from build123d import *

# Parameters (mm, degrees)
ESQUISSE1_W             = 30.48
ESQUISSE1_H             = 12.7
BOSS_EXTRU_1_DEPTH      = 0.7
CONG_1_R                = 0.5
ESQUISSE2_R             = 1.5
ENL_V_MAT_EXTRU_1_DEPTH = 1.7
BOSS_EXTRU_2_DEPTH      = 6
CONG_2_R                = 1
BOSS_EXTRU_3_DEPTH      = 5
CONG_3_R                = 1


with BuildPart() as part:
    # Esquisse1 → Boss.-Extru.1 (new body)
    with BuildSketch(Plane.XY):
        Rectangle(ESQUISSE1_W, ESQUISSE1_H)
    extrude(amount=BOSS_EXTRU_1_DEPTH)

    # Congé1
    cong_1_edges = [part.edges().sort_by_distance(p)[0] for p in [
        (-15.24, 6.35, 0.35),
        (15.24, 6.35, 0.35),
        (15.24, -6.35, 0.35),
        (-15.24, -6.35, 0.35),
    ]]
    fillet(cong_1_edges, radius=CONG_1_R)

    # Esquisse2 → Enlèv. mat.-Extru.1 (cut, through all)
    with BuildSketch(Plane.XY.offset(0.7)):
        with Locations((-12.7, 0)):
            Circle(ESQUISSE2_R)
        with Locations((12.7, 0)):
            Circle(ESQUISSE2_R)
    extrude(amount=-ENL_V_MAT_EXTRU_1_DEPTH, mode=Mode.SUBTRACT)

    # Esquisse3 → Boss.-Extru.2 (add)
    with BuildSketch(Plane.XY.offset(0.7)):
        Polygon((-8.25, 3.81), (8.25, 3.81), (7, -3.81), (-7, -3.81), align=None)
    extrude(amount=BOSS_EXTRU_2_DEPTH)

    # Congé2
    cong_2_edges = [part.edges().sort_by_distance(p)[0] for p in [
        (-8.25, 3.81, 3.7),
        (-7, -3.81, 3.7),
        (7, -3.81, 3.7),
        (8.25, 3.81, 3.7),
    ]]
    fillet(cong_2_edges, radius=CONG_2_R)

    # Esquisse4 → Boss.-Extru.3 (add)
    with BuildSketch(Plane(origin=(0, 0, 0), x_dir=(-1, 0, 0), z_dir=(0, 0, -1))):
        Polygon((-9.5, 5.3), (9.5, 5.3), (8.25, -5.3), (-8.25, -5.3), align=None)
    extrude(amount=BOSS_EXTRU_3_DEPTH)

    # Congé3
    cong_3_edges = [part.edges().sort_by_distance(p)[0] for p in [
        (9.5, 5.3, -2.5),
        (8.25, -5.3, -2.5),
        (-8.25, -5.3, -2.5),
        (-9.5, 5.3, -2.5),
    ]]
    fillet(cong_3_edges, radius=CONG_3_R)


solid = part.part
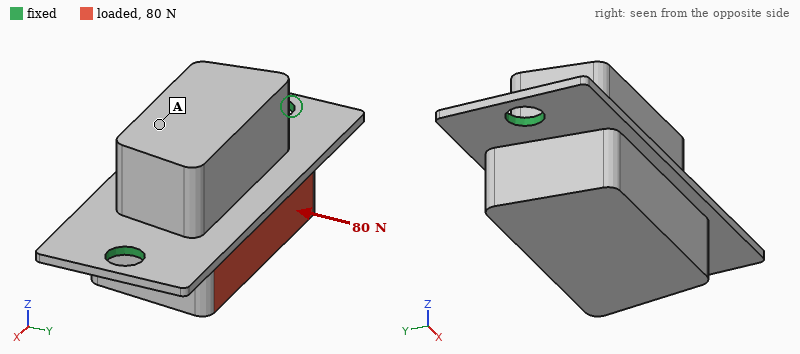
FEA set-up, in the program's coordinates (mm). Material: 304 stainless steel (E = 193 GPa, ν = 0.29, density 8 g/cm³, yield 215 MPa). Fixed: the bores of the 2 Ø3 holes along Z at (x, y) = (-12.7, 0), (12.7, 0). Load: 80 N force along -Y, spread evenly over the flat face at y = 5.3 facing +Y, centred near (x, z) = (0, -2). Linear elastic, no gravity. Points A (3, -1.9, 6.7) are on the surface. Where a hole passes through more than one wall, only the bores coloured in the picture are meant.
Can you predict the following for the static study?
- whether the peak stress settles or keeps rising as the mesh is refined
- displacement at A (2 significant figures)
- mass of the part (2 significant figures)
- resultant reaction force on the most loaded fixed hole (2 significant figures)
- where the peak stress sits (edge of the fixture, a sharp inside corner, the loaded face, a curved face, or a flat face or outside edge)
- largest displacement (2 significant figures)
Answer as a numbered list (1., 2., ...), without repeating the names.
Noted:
1. keeps rising
2. 12 µm
3. 15 g
4. 40 N
5. edge of the fixture
6. 14 µm
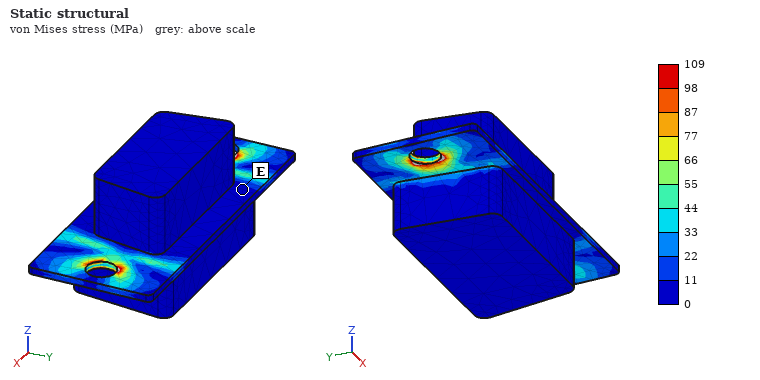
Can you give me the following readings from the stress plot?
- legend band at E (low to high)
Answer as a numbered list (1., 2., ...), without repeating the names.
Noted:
1. 0 to 11 MPa
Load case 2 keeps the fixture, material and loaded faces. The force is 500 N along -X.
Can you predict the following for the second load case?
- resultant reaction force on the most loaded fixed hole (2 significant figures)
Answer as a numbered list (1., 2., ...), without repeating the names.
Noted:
1. 280 N
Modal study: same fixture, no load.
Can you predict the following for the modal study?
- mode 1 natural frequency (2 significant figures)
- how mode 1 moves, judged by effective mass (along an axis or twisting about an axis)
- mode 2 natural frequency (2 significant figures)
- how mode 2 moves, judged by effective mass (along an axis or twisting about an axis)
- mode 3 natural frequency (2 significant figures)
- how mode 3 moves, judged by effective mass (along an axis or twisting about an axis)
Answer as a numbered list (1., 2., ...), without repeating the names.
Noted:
1. 3400 Hz
2. twisting about X
3. 7000 Hz
4. along Z
5. 12 kHz
6. twisting about Y
